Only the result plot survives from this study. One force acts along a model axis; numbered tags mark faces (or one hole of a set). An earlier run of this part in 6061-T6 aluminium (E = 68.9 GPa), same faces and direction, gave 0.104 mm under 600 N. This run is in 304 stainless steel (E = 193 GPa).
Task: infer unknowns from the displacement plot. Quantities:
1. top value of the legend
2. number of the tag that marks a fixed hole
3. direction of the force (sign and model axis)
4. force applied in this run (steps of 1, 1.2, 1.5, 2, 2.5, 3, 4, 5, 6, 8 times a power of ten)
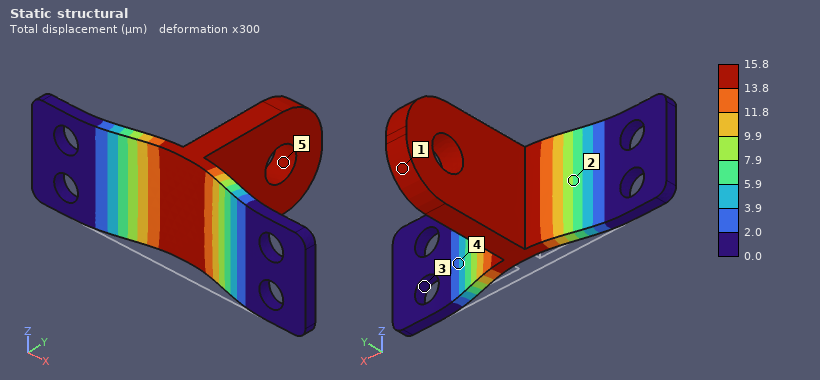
15.8 µm
3
+Y
250 N
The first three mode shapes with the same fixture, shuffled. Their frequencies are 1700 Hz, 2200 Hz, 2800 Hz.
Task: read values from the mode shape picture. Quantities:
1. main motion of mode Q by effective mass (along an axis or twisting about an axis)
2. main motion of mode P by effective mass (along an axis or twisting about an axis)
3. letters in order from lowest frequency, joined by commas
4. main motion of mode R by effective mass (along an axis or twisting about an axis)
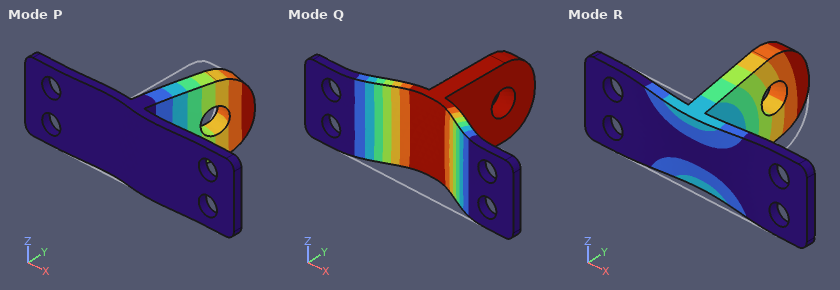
along Y
along X
R, P, Q
along Z
